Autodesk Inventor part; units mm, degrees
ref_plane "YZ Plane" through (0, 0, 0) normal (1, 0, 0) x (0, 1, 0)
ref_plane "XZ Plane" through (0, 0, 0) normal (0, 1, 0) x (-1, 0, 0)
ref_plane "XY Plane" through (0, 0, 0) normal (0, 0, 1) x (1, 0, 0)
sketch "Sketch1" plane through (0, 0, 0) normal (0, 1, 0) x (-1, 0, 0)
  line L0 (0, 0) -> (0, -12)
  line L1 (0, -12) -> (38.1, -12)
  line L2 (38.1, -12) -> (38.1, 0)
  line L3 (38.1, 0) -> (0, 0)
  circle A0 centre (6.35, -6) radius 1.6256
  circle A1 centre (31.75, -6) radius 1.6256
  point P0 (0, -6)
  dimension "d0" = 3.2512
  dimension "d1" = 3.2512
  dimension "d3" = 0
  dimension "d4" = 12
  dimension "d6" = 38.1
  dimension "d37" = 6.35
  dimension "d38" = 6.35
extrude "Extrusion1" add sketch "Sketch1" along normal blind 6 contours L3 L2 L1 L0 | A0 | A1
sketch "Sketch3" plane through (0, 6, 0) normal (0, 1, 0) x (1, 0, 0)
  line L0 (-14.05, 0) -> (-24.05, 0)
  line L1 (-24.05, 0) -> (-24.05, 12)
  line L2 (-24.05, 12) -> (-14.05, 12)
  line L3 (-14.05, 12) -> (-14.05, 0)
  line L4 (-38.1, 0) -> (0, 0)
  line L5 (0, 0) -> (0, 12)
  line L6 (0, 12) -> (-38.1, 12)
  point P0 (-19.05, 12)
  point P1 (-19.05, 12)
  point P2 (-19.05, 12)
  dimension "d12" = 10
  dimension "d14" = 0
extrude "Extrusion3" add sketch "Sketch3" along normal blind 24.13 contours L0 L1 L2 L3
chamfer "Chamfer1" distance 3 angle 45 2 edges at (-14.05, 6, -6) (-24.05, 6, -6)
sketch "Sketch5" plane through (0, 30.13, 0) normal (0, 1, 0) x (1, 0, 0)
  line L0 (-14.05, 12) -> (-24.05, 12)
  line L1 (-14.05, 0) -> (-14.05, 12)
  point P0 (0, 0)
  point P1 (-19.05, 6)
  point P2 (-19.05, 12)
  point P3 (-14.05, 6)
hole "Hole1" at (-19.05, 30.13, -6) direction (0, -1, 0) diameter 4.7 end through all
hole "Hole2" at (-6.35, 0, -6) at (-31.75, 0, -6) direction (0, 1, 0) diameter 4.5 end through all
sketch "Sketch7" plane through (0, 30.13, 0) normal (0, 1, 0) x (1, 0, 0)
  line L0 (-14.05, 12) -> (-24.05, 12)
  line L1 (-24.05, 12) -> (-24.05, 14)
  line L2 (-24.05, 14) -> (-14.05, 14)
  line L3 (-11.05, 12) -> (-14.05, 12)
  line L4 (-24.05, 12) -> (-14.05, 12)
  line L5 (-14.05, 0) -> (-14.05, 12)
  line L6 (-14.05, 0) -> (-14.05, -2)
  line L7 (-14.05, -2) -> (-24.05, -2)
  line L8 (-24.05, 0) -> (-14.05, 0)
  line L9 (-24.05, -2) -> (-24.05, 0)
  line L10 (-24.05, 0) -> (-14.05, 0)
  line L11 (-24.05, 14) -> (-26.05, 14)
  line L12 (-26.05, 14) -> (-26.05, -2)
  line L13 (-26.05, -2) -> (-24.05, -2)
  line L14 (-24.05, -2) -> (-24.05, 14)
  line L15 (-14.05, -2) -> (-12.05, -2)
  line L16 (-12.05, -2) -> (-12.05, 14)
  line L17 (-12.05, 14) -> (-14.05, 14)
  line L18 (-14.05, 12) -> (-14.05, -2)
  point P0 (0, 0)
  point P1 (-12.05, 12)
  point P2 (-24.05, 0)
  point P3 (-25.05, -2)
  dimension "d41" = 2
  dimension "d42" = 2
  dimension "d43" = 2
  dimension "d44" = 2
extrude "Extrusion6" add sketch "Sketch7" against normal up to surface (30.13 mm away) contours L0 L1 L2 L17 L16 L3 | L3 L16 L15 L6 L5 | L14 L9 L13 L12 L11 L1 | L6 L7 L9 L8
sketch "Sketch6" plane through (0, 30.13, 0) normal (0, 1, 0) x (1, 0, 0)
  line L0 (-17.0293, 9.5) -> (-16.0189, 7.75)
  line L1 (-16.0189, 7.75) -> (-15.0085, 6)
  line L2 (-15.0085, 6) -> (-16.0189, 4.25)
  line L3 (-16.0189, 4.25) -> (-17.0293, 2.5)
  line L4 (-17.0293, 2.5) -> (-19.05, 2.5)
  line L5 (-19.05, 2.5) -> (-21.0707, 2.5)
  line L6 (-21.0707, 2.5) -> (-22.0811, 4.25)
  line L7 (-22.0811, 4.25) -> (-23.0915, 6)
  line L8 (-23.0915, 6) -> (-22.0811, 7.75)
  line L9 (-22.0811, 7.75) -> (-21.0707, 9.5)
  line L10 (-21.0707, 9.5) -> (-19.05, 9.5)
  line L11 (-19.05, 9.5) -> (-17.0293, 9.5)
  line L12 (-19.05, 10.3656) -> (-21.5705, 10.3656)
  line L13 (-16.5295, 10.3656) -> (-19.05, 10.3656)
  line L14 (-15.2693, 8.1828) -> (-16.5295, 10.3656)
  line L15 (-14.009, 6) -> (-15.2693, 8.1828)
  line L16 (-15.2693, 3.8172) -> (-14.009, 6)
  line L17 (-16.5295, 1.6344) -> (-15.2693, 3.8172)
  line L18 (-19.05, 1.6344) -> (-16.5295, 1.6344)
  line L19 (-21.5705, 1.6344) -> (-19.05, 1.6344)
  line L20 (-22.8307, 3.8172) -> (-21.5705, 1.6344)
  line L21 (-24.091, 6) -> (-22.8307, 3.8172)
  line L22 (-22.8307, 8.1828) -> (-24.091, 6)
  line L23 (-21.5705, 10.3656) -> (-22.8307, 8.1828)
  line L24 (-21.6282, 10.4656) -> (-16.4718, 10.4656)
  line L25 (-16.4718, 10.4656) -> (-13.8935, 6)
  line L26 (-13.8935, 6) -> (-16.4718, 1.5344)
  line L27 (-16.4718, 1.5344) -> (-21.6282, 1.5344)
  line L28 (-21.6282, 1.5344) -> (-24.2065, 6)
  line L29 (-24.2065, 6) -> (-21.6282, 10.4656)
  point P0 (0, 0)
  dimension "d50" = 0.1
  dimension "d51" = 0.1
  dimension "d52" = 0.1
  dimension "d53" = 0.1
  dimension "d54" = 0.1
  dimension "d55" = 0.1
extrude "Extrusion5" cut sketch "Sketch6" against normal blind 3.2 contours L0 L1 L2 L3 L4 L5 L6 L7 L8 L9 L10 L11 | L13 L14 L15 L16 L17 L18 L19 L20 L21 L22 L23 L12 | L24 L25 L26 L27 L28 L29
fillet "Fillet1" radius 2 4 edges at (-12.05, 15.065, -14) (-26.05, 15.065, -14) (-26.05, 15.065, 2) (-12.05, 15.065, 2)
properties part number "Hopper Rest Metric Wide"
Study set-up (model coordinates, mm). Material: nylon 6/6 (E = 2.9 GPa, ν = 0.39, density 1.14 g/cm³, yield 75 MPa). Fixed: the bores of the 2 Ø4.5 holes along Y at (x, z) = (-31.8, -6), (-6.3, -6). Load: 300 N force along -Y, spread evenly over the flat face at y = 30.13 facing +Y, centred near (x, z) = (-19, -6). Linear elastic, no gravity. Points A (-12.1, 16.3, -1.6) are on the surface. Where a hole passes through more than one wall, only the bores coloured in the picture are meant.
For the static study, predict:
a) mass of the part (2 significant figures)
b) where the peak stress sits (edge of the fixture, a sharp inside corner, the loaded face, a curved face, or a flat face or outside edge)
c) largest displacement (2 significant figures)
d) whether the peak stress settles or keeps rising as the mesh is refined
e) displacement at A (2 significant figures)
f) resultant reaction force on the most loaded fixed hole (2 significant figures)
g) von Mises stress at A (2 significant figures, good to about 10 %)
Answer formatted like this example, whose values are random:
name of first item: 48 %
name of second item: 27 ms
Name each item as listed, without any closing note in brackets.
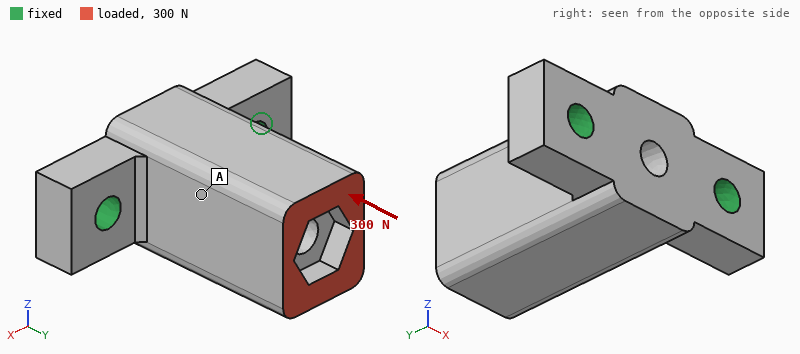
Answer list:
mass of the part: 8.6 g
where the peak stress sits: edge of the fixture
largest displacement: 35 µm
whether the peak stress settles or keeps rising as the mesh is refined: keeps rising
displacement at A: 26 µm
resultant reaction force on the most loaded fixed hole: 160 N
von Mises stress at A: 1.4 MPa
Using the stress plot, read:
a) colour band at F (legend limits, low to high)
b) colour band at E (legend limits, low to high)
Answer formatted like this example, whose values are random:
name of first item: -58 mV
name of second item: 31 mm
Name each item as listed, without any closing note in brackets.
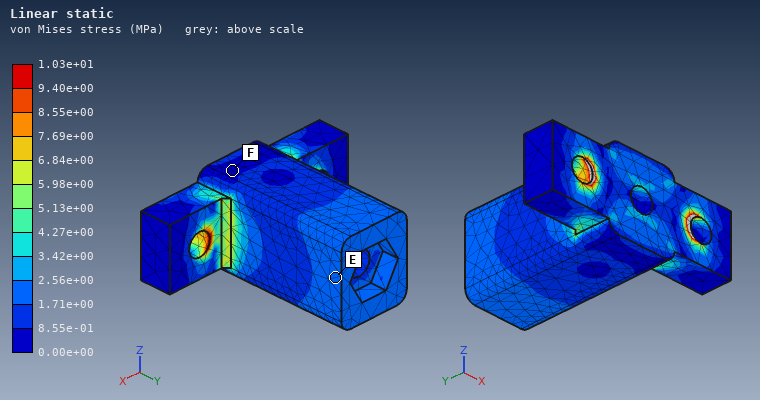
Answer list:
colour band at F: 0.00e+00 to 8.55e-01 MPa
colour band at E: 1.71e+00 to 2.56e+00 MPa
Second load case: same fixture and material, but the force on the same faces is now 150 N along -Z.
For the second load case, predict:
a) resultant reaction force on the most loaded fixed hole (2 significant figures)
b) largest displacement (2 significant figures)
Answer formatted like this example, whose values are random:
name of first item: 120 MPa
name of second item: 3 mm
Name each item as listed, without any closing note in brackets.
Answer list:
resultant reaction force on the most loaded fixed hole: 75 N
largest displacement: 0.56 mm
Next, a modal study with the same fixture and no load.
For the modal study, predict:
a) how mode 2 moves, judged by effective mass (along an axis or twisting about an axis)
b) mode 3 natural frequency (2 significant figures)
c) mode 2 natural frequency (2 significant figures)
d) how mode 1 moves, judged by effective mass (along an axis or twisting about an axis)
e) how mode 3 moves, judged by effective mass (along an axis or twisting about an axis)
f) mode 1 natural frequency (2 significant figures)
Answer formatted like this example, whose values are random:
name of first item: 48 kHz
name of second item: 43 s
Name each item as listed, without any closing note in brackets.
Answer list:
how mode 2 moves, judged by effective mass: along X
mode 3 natural frequency: 6900 Hz
mode 2 natural frequency: 3700 Hz
how mode 1 moves, judged by effective mass: along Z
how mode 3 moves, judged by effective mass: along Y
mode 1 natural frequency: 1900 Hz
